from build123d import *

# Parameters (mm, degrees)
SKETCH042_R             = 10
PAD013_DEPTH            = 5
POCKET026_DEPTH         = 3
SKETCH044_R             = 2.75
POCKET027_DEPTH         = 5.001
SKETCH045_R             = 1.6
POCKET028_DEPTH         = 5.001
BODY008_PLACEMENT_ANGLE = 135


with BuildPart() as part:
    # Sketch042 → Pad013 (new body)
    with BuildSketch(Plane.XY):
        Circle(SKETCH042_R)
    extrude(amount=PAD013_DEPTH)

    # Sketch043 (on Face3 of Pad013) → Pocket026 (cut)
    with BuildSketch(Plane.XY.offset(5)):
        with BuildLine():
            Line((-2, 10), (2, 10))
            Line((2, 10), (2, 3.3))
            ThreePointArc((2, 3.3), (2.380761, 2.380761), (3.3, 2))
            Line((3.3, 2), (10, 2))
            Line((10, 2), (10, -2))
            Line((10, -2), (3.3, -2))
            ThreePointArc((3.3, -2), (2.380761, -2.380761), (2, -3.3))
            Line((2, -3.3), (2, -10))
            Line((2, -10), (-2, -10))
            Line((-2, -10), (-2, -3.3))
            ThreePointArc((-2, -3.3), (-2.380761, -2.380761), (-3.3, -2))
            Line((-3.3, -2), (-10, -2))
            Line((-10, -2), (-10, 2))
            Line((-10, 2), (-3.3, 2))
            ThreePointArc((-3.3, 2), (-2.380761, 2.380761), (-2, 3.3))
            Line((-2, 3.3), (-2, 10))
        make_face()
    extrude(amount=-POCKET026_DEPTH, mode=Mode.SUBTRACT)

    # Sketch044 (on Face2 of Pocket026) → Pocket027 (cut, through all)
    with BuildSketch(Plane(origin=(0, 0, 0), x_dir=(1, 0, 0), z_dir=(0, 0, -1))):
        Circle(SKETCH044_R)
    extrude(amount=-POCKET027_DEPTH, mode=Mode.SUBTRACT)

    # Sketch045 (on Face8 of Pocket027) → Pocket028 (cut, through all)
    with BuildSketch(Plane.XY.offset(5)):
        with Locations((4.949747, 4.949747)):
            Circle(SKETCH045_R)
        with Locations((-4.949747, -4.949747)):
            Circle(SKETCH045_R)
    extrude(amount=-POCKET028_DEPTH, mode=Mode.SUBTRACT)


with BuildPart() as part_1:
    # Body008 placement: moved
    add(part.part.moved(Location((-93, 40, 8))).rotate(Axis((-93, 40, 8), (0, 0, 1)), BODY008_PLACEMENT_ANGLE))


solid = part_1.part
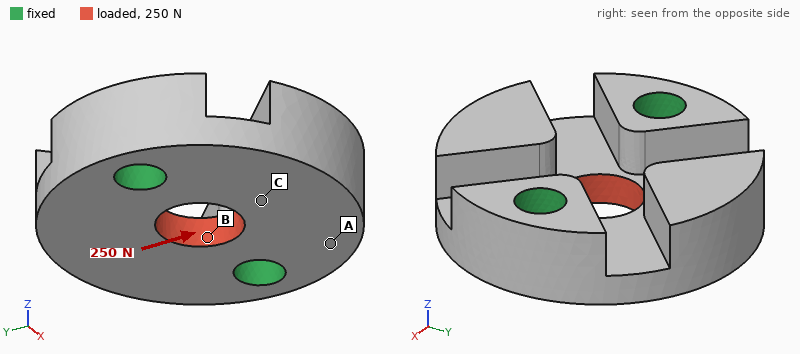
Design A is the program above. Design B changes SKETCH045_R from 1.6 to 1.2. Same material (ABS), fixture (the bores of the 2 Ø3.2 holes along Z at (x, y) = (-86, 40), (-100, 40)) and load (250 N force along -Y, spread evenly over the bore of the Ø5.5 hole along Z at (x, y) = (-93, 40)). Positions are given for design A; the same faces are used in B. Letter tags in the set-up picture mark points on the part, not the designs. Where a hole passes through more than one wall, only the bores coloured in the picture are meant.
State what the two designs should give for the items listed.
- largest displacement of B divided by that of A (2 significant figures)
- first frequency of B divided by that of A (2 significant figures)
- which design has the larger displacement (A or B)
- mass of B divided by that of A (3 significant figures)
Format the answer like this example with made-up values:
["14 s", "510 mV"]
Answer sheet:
["1.1", "0.97", "B", "1.03"]
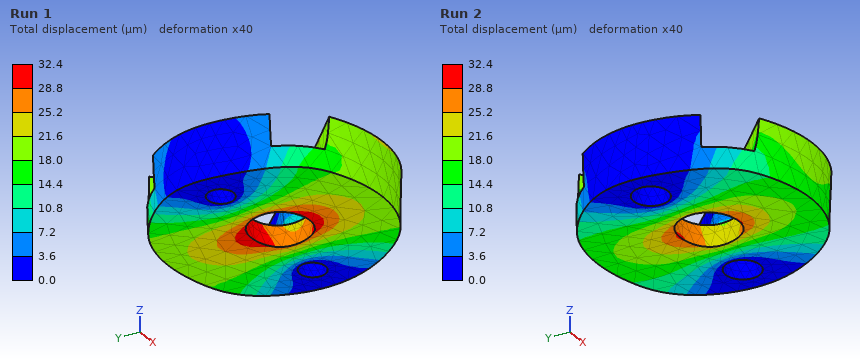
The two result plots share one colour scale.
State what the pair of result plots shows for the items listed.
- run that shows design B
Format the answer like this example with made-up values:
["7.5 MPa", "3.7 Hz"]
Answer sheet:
["Run 1"]
